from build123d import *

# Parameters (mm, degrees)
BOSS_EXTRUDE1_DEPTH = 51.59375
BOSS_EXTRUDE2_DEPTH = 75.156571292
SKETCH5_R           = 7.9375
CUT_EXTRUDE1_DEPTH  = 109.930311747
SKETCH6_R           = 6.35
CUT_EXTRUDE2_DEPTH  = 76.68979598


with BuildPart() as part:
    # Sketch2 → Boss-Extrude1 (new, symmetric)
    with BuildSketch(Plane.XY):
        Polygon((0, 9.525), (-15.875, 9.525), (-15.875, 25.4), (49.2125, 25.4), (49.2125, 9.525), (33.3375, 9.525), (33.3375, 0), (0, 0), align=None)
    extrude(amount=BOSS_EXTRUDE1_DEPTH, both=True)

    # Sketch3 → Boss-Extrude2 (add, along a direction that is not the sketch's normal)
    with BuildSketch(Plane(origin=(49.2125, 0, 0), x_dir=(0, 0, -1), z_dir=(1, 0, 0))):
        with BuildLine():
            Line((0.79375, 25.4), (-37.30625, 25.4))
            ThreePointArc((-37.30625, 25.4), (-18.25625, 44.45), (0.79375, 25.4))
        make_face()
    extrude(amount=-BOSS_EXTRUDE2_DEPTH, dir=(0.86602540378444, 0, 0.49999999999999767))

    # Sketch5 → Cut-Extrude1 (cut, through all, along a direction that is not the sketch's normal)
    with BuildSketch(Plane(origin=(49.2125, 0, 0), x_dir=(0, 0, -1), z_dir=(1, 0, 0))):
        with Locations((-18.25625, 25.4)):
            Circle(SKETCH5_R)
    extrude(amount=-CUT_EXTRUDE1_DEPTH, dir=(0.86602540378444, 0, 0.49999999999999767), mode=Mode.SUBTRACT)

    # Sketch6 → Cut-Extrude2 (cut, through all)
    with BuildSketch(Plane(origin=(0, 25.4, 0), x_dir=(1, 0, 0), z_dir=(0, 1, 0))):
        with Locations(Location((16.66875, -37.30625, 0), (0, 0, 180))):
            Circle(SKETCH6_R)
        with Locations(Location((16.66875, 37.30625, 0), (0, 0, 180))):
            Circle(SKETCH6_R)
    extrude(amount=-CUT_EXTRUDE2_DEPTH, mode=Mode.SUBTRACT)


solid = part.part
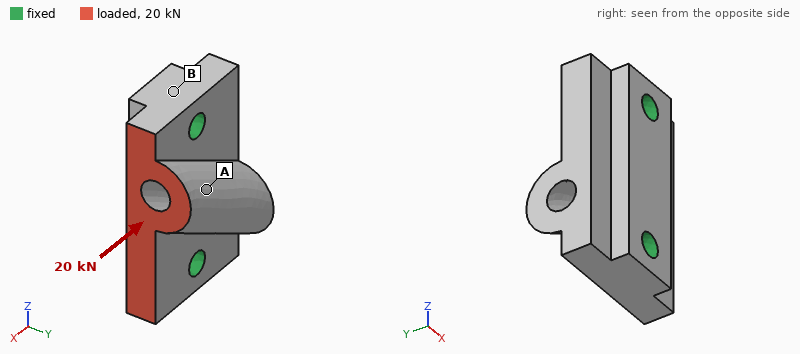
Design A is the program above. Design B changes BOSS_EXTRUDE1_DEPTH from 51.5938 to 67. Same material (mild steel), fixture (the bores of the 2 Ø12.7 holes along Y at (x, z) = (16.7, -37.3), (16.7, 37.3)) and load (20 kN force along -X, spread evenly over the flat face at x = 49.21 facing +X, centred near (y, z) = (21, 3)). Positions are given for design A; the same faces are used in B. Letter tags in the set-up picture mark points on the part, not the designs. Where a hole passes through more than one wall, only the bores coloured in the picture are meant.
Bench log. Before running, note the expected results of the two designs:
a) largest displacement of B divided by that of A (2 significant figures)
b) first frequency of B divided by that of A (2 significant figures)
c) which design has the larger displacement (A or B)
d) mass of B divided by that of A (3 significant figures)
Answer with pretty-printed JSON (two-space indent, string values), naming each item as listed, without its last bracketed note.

{
  "largest displacement of B divided by that of A": "0.79",
  "first frequency of B divided by that of A": "1.0",
  "which design has the larger displacement": "A",
  "mass of B divided by that of A": "1.26"
}
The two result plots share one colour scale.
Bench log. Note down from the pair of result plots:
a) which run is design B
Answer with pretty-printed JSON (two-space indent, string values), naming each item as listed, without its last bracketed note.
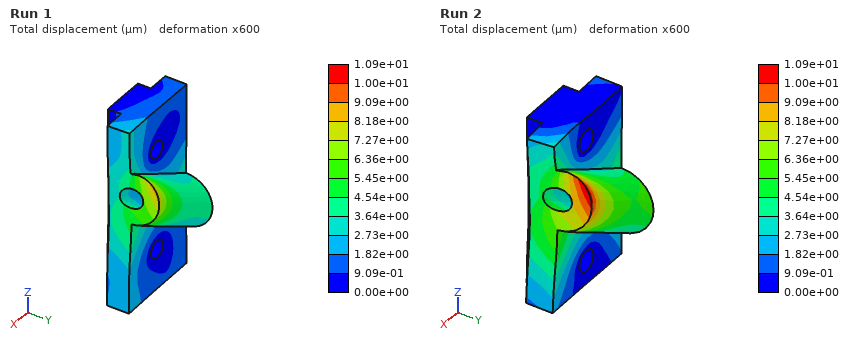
{
  "which run is design B": "Run 1"
}
